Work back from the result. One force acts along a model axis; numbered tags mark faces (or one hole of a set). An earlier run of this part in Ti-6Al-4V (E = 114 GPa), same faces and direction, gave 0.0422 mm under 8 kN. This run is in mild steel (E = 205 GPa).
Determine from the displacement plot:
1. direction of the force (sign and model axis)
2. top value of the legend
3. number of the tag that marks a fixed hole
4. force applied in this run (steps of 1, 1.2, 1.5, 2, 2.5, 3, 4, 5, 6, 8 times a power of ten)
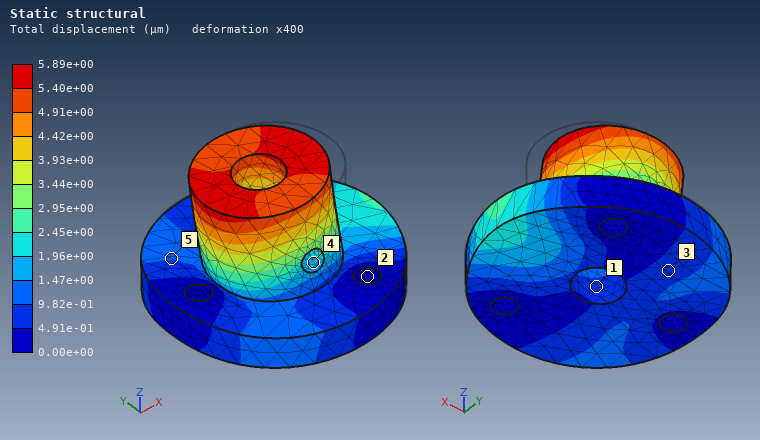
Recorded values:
-X
5.89e+00 µm
2
2 kN
